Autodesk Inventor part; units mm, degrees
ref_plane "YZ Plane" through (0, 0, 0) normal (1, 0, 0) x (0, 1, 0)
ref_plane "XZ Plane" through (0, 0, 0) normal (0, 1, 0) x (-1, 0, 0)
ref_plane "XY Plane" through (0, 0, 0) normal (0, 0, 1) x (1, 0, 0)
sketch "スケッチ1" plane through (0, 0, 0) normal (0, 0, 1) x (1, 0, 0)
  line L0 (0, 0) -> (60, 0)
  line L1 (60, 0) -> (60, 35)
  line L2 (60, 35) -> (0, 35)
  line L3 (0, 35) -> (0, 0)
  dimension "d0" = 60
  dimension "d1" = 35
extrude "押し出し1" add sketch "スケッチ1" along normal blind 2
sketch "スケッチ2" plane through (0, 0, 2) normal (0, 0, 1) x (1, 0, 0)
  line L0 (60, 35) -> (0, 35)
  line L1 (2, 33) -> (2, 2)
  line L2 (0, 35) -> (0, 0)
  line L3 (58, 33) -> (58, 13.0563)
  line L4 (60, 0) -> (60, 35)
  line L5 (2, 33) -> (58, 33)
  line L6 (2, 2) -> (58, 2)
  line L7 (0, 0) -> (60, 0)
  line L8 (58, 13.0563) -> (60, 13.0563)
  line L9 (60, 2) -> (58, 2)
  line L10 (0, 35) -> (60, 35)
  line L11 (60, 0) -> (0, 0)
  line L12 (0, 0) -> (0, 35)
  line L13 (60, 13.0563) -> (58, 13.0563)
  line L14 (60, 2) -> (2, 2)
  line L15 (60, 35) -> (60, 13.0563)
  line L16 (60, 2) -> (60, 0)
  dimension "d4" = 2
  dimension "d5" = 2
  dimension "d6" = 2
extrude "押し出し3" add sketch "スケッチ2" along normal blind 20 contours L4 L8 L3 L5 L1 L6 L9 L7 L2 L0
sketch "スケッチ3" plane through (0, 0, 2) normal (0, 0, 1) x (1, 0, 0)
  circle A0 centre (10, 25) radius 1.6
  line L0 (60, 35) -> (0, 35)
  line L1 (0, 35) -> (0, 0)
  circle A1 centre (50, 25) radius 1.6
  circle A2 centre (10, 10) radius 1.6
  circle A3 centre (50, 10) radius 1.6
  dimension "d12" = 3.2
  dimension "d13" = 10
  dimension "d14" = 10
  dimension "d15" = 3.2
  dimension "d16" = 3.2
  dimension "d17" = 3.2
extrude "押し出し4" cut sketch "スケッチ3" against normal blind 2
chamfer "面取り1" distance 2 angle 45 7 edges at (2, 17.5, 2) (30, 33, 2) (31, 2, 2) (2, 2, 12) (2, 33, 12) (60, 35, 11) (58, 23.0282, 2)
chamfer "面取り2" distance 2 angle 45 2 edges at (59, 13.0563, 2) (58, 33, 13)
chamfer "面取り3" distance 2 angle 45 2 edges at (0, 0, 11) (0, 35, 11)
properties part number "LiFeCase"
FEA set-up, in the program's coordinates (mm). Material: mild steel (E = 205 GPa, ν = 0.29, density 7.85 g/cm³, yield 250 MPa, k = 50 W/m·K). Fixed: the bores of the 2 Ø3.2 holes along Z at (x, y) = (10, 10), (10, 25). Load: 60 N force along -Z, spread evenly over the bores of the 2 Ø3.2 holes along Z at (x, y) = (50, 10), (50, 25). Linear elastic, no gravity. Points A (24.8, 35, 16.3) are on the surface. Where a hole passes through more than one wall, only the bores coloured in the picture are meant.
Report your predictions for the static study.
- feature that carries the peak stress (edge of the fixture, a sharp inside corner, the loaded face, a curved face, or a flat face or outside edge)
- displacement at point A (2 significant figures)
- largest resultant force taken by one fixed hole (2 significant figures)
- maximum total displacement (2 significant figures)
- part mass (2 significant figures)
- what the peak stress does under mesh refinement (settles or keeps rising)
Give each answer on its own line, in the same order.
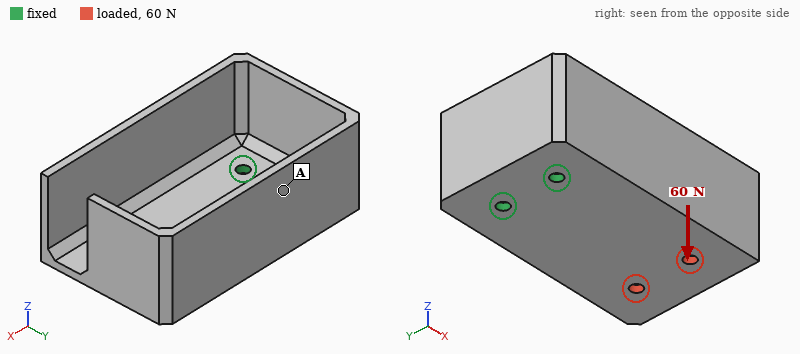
edge of the fixture
26 µm
31 N
65 µm
89 g
keeps rising
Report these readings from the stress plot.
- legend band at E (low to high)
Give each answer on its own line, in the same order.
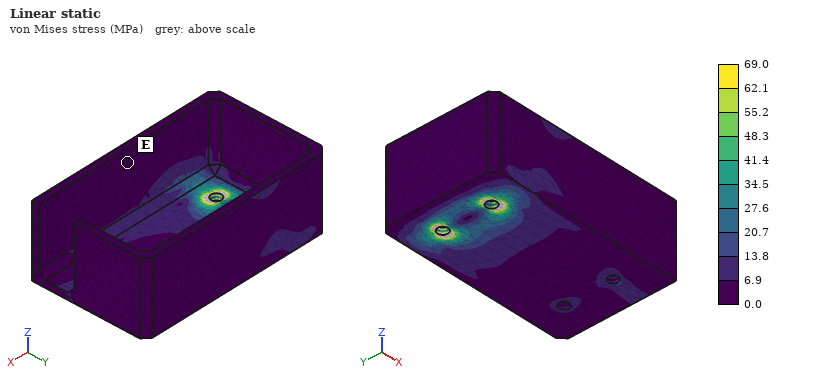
0.0 to 6.9 MPa
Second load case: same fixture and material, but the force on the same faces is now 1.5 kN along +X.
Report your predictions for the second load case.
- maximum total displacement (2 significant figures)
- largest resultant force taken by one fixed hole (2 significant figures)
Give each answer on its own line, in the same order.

6.7 µm
750 N
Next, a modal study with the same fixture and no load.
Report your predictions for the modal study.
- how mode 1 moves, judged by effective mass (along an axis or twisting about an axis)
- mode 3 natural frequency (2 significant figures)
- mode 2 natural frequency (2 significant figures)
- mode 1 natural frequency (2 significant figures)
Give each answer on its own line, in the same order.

along Z
2900 Hz
1500 Hz
830 Hz
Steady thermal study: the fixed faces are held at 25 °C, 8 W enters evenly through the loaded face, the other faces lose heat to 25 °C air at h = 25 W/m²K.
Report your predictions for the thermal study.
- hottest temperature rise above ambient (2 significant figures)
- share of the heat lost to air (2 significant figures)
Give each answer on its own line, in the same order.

42 K
55 %
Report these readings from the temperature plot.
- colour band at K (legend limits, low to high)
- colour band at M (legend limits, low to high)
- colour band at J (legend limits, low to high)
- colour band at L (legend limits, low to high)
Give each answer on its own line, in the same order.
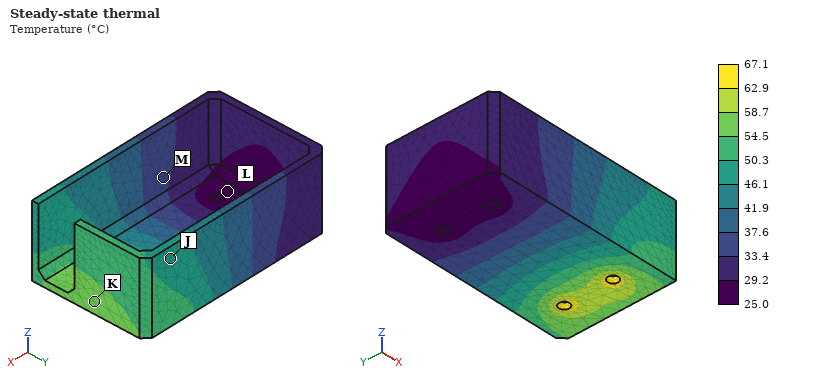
54.5 to 58.7 °C
33.4 to 37.6 °C
46.1 to 50.3 °C
25.0 to 29.2 °C
